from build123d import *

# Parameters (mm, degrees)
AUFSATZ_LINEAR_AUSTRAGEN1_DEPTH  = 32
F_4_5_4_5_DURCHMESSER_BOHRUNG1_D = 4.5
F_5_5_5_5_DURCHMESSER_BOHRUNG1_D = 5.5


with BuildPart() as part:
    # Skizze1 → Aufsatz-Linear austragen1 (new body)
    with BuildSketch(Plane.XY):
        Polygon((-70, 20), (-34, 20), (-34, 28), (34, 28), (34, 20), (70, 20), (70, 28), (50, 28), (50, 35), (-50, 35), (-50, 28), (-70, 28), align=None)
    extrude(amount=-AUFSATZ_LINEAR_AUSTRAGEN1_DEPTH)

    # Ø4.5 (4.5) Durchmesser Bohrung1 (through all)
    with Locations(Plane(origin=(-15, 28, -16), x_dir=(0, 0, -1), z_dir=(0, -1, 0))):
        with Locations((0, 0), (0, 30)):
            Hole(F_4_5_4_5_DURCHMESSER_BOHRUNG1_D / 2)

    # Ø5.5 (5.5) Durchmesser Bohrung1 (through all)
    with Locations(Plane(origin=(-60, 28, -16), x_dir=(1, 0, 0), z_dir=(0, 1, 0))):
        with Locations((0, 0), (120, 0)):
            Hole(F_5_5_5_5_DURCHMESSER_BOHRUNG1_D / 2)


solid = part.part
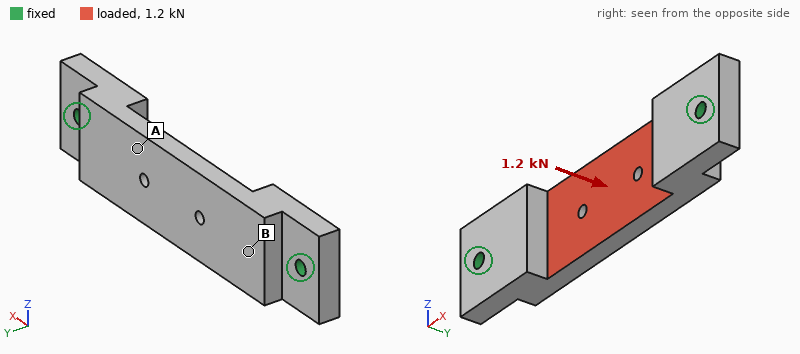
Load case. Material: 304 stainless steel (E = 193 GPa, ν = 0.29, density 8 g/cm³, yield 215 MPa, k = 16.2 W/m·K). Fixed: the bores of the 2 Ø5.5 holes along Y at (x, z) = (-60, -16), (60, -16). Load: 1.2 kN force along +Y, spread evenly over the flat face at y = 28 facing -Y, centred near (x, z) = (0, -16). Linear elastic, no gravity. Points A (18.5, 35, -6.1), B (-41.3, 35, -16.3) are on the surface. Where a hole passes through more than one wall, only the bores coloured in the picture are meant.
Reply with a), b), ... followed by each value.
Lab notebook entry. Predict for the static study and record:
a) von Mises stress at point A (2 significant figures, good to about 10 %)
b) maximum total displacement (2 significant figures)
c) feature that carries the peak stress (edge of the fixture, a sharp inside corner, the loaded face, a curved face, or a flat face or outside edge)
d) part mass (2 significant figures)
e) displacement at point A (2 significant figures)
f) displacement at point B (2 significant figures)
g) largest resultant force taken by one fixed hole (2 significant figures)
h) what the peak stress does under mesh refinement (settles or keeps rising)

a) 17 MPa
b) 21 µm
c) edge of the fixture
d) 320 g
e) 15 µm
f) 5.5 µm
g) 1.7 kN
h) keeps rising
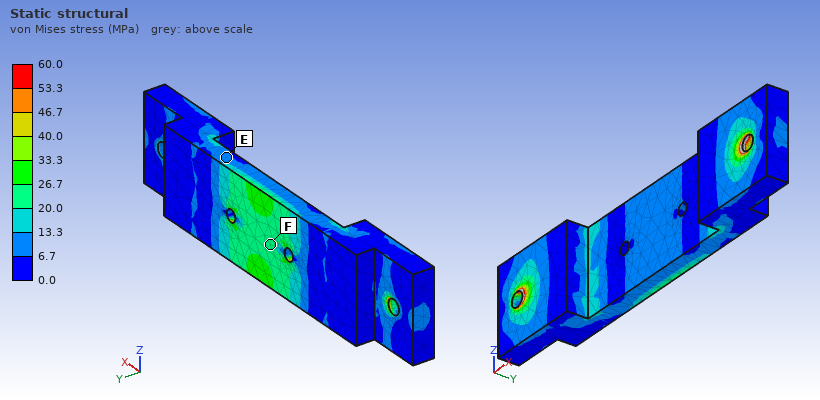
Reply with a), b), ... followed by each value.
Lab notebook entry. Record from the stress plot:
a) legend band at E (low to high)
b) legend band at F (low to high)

a) 6.7 to 13.3 MPa
b) 20.0 to 26.7 MPa
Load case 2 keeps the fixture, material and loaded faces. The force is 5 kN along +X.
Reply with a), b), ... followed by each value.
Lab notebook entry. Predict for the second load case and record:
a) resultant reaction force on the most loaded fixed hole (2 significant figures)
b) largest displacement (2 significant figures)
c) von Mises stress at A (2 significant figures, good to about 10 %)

a) 2.5 kN
b) 13 µm
c) 14 MPa
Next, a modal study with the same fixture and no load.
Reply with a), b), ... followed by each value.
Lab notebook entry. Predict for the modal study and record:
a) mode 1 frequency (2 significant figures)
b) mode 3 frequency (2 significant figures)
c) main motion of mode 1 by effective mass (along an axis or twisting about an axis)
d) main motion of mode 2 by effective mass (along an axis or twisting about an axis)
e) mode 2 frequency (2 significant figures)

a) 3700 Hz
b) 5600 Hz
c) along Y
d) along Z
e) 4600 Hz
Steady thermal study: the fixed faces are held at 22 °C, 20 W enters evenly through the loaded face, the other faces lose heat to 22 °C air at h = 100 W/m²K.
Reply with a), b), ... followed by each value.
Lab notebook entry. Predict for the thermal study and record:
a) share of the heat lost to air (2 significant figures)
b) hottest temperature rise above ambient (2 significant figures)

a) 79 %
b) 41 K
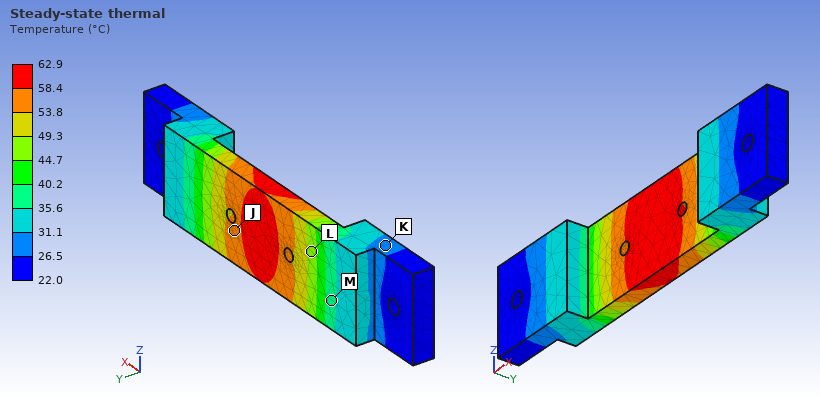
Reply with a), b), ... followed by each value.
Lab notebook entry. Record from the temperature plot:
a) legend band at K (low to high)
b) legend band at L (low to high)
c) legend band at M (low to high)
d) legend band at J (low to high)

a) 26.5 to 31.1 °C
b) 44.7 to 49.3 °C
c) 35.6 to 40.2 °C
d) 53.8 to 58.4 °C
